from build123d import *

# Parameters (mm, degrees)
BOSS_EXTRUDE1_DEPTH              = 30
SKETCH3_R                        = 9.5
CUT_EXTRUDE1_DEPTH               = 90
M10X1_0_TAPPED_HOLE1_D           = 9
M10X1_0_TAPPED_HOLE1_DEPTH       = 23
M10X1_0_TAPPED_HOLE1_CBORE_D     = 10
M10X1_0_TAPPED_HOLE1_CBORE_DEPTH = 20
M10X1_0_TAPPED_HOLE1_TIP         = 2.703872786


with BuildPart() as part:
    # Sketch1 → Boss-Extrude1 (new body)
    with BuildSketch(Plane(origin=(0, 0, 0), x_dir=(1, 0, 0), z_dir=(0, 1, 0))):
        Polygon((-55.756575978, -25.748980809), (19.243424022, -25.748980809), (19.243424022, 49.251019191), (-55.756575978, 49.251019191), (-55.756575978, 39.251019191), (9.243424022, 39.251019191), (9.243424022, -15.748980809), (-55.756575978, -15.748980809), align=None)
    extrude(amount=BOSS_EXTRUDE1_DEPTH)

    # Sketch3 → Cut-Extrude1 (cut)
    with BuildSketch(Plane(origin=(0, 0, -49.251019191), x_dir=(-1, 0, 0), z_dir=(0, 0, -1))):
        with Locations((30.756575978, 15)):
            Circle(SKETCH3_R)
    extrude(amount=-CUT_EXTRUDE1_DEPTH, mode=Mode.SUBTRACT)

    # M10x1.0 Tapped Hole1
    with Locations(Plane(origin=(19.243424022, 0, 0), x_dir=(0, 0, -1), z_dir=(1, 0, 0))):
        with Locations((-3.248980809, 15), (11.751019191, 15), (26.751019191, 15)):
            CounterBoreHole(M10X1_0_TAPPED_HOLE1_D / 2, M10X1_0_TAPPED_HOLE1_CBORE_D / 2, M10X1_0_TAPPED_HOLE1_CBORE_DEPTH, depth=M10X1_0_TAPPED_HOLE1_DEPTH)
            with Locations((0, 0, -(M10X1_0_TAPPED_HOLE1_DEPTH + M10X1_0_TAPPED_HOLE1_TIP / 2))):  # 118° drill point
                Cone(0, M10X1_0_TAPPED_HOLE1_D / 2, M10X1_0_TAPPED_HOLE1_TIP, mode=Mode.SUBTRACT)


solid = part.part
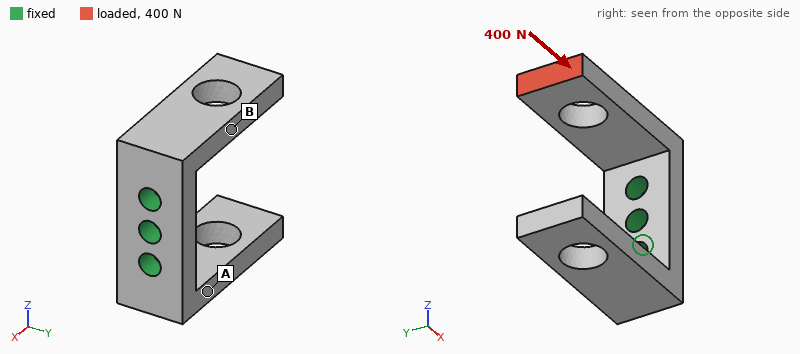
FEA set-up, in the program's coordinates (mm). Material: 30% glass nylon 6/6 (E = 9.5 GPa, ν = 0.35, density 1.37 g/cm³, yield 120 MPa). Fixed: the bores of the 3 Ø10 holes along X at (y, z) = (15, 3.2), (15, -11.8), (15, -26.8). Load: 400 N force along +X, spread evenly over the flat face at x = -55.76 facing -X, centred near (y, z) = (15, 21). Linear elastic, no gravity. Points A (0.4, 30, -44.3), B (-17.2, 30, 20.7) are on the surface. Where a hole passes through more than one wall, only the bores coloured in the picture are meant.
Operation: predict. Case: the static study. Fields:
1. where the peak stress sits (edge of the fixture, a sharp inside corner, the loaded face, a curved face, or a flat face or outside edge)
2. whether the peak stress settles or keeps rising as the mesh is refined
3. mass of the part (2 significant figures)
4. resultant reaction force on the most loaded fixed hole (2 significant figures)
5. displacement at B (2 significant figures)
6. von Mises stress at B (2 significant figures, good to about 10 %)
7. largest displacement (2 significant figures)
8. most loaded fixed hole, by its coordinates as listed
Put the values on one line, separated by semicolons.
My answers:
edge of the fixture; keeps rising; 73 g; 460 N; 0.073 mm; 3.1 MPa; 0.16 mm; (15, 3.2)
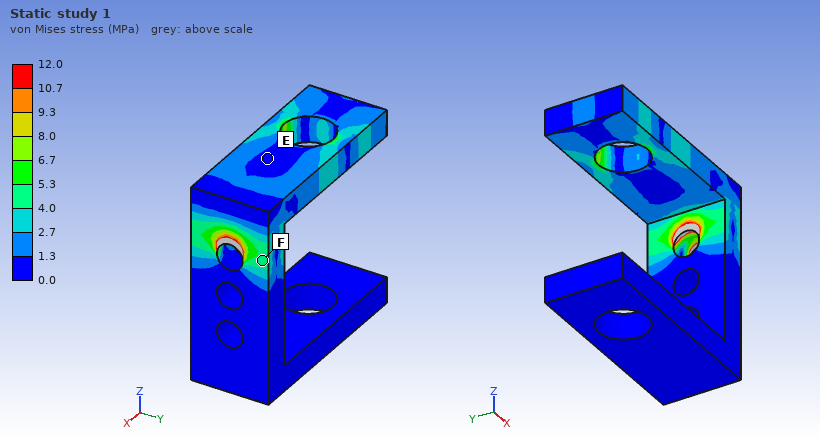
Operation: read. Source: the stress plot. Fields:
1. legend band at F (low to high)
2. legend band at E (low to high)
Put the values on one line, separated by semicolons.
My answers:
4.0 to 5.3 MPa; 0.0 to 1.3 MPa
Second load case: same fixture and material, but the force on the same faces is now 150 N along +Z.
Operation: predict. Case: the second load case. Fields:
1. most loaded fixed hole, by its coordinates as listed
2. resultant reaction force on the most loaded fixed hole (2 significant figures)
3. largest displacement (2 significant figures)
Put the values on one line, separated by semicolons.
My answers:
(15, 3.2); 190 N; 1.2 mm
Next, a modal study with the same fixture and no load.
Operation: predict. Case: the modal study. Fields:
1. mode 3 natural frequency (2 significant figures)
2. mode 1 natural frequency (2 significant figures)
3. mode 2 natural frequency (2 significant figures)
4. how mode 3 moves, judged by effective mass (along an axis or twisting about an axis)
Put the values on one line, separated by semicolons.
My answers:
1100 Hz; 710 Hz; 710 Hz; twisting about X
